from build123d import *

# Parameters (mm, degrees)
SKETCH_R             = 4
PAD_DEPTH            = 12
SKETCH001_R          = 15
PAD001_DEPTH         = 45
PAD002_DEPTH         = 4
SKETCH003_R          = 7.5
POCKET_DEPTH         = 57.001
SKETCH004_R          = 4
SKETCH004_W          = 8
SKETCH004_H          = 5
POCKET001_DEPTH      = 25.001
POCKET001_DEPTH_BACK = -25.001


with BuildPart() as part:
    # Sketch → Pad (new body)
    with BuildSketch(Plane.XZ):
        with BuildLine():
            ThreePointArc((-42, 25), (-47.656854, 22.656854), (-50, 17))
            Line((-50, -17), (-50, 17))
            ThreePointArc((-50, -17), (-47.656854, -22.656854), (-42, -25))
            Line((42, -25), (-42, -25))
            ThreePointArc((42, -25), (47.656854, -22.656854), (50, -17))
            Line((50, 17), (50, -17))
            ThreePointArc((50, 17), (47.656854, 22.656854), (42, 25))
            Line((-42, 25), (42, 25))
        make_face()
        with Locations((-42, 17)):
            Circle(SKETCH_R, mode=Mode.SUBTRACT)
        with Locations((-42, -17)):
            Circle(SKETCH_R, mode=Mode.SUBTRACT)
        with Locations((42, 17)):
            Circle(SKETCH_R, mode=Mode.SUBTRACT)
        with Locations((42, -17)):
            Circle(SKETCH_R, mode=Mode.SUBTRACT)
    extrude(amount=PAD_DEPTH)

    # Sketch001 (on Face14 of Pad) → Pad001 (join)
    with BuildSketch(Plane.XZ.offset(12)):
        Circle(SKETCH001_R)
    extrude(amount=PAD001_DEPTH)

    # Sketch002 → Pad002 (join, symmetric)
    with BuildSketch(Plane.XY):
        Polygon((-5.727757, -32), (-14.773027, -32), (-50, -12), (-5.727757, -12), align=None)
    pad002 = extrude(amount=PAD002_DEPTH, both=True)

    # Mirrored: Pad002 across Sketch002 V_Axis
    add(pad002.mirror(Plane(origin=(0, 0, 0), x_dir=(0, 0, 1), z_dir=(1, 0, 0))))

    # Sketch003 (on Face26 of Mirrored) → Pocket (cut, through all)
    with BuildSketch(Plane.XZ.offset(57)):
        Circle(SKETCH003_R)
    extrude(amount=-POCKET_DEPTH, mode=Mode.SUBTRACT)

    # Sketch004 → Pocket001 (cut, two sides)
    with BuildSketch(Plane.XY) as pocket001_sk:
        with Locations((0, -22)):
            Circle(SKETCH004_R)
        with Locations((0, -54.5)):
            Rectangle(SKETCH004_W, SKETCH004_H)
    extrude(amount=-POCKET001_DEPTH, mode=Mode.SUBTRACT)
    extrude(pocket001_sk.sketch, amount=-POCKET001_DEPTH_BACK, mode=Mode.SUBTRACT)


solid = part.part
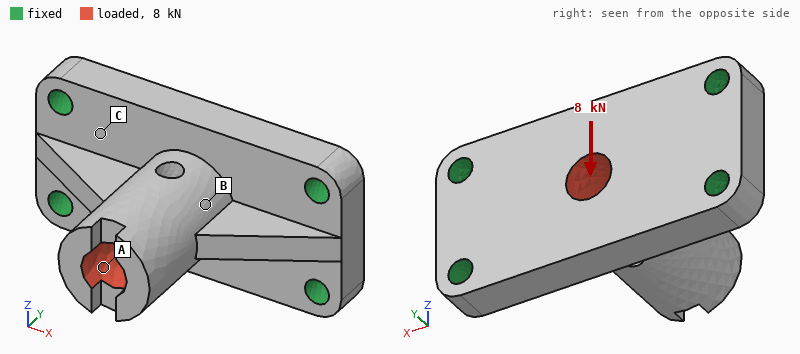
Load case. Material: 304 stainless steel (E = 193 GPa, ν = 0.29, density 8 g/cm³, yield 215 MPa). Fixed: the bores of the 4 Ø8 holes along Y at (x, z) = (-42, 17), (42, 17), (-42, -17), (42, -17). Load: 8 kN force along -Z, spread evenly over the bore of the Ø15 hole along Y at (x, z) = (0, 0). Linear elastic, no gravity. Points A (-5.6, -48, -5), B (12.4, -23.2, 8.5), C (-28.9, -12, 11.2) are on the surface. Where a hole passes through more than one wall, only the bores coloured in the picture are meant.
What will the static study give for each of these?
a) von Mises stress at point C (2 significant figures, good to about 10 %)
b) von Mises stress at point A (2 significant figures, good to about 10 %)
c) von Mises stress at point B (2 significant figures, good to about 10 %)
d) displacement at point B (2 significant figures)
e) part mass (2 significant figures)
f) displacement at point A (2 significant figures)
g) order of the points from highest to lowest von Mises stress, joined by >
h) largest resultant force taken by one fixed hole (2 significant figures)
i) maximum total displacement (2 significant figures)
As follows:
45 MPa
9.8 MPa
25 MPa
21 µm
660 g
51 µm
C > B > A
3.8 kN
64 µm
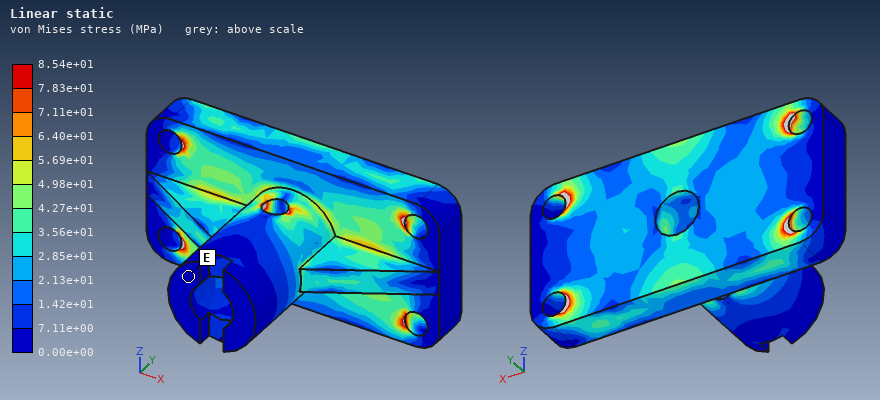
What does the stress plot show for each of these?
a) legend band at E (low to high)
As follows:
0.00e+00 to 7.11e+00 MPa
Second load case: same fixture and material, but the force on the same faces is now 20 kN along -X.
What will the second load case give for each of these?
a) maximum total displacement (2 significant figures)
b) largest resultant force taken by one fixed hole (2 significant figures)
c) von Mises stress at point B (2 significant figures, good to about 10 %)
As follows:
34 µm
6.0 kN
31 MPa
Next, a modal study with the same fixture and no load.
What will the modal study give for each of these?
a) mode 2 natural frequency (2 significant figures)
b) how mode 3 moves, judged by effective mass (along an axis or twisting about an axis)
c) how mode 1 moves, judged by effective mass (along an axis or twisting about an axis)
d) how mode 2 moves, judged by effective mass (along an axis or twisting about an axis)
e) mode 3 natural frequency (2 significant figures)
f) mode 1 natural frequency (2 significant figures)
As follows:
7400 Hz
along X
along Z
along Y
9300 Hz
4300 Hz
